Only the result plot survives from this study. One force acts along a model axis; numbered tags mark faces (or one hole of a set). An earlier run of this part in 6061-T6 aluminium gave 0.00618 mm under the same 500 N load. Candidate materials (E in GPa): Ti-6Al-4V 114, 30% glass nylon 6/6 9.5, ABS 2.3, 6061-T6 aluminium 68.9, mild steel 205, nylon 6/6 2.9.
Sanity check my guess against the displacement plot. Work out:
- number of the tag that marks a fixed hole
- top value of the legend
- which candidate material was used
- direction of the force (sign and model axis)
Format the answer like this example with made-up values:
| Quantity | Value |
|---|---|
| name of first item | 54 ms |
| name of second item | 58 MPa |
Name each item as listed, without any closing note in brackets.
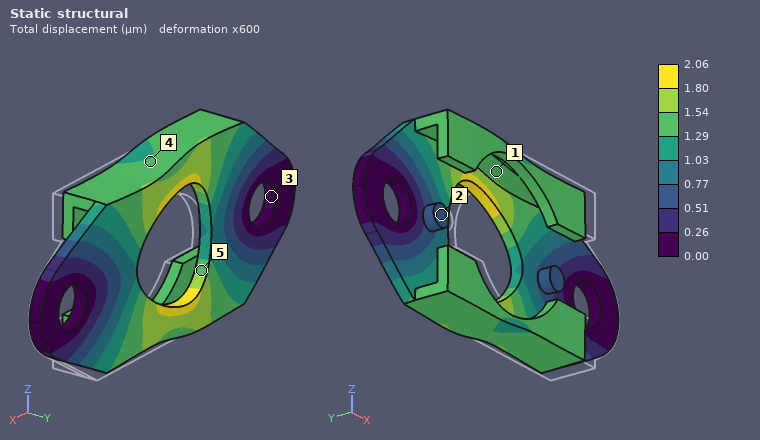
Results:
| Quantity | Value |
|---|---|
| number of the tag that marks a fixed hole | 3 |
| top value of the legend | 2.06 µm |
| which candidate material was used | mild steel |
| direction of the force | -X |
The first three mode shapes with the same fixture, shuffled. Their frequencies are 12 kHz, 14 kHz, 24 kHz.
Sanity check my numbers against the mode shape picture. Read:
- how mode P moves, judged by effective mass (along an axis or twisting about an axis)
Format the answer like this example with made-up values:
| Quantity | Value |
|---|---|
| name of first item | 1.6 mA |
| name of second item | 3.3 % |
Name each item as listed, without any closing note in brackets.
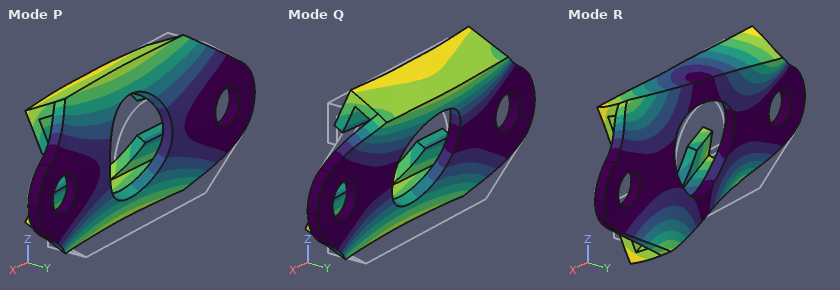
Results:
| Quantity | Value |
|---|---|
| how mode P moves, judged by effective mass | along Y |
